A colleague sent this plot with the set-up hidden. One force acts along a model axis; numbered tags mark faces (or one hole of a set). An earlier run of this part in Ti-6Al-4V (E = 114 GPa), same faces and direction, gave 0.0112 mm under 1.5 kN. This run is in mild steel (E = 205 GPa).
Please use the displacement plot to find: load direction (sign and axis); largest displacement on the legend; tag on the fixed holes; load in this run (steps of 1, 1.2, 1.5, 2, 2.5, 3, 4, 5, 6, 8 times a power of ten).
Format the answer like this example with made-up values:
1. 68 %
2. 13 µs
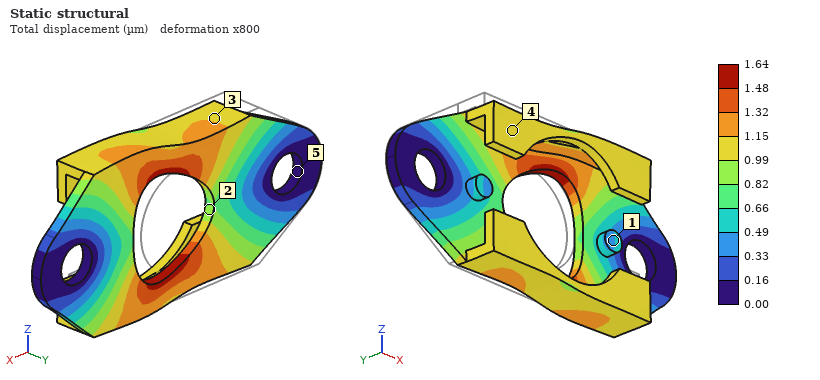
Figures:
1. +X
2. 1.64 µm
3. 5
4. 400 N
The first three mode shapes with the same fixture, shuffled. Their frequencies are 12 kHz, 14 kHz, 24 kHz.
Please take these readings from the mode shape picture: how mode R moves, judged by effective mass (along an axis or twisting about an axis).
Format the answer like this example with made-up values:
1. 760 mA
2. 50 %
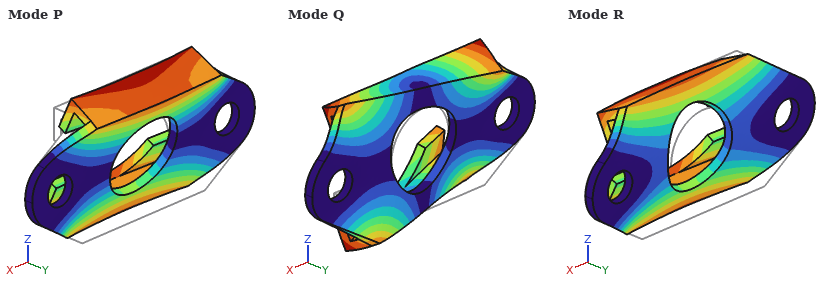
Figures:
1. along Y
